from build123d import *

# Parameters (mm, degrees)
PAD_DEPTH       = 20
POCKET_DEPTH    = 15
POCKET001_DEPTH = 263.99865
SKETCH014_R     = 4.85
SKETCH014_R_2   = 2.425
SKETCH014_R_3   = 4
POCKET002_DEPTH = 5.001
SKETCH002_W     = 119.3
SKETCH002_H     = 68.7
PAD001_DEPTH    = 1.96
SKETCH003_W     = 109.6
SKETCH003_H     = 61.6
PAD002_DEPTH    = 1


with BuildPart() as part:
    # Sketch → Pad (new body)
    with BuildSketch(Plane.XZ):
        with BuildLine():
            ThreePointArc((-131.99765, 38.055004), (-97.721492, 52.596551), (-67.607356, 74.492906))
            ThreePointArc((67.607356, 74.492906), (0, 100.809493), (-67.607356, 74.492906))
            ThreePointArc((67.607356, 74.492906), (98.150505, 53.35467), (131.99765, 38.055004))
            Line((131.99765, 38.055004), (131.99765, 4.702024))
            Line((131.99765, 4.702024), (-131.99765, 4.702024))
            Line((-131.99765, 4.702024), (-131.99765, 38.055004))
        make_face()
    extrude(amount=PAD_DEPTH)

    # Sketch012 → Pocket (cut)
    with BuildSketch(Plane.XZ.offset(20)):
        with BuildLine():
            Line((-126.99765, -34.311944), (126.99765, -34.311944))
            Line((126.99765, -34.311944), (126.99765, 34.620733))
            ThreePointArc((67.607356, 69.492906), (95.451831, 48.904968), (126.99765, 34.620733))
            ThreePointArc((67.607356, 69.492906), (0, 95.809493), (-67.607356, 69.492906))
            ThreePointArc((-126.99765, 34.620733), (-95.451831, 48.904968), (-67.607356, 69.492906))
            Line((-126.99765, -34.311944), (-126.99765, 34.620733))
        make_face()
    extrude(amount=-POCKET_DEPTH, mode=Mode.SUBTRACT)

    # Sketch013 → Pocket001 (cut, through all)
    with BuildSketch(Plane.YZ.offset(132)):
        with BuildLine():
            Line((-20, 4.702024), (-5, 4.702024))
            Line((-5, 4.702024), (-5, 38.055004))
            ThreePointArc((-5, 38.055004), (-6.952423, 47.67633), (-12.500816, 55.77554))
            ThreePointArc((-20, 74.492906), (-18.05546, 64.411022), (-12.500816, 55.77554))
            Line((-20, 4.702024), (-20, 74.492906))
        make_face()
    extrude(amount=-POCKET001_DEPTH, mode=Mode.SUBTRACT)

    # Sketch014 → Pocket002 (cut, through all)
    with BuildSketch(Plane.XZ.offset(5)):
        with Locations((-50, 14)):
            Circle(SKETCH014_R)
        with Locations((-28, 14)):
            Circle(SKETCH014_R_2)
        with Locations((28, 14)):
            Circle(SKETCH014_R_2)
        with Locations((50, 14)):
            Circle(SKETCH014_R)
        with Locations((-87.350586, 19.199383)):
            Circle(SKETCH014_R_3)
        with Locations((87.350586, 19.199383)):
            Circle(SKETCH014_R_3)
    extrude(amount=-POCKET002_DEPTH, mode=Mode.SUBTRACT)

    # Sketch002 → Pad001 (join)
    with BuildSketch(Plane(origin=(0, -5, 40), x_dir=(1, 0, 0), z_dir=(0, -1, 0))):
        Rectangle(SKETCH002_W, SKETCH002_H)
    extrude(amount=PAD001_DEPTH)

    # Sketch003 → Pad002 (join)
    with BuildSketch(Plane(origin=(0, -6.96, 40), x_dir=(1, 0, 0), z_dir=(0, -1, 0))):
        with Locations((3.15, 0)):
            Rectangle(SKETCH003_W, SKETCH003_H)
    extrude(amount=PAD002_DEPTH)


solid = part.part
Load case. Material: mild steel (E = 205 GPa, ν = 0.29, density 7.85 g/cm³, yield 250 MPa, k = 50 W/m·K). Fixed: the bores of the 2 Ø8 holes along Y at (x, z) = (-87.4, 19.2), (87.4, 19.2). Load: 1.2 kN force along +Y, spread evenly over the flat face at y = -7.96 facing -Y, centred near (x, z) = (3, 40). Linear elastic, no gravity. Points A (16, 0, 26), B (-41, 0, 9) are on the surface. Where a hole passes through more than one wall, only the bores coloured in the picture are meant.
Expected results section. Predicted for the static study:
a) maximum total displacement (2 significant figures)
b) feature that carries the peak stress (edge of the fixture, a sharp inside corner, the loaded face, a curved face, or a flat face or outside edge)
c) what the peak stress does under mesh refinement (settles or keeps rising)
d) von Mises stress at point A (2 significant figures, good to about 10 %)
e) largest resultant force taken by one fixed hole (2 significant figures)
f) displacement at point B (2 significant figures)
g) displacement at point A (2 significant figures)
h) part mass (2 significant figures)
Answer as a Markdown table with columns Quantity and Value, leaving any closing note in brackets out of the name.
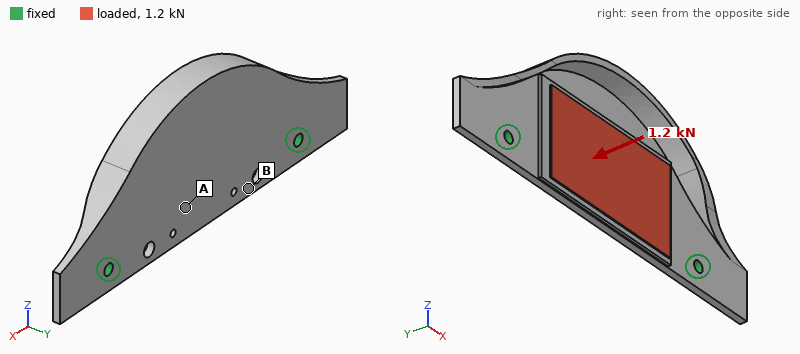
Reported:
| Quantity | Value |
|---|---|
| maximum total displacement | 0.18 mm |
| feature that carries the peak stress | edge of the fixture |
| what the peak stress does under mesh refinement | keeps rising |
| von Mises stress at point A | 16 MPa |
| largest resultant force taken by one fixed hole | 910 N |
| displacement at point B | 0.031 mm |
| displacement at point A | 0.066 mm |
| part mass | 990 g |
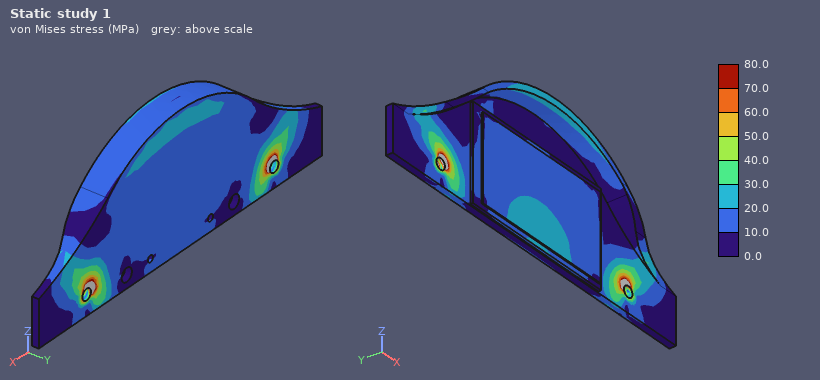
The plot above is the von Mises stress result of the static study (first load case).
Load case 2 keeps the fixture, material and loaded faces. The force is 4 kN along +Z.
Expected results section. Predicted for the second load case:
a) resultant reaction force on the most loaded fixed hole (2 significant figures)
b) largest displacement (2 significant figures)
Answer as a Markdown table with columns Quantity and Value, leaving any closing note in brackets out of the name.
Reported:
| Quantity | Value |
|---|---|
| resultant reaction force on the most loaded fixed hole | 2.5 kN |
| largest displacement | 0.16 mm |
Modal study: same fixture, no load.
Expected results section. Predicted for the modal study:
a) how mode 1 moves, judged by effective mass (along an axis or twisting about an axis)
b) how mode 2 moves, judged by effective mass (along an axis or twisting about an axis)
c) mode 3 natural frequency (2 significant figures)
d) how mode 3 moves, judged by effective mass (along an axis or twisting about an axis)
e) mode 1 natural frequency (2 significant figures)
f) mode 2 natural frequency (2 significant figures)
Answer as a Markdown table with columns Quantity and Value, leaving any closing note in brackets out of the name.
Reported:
| Quantity | Value |
|---|---|
| how mode 1 moves, judged by effective mass | along Y |
| how mode 2 moves, judged by effective mass | along Y |
| mode 3 natural frequency | 1900 Hz |
| how mode 3 moves, judged by effective mass | twisting about Z |
| mode 1 natural frequency | 480 Hz |
| mode 2 natural frequency | 1300 Hz |
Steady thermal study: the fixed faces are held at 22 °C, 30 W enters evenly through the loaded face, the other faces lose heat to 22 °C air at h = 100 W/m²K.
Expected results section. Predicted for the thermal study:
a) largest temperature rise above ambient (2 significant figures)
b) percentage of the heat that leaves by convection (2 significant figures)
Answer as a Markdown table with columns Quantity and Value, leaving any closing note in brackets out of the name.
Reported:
| Quantity | Value |
|---|---|
| largest temperature rise above ambient | 16 K |
| percentage of the heat that leaves by convection | 85 % |
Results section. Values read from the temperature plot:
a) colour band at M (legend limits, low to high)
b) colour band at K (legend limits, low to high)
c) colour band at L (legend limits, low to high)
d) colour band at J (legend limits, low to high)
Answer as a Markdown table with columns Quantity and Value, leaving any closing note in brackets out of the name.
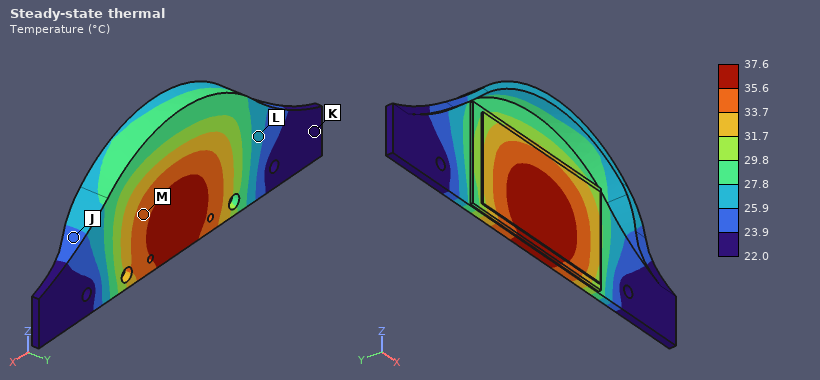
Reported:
| Quantity | Value |
|---|---|
| colour band at M | 33.7 to 35.6 °C |
| colour band at K | 22.0 to 23.9 °C |
| colour band at L | 25.9 to 27.8 °C |
| colour band at J | 23.9 to 25.9 °C |
